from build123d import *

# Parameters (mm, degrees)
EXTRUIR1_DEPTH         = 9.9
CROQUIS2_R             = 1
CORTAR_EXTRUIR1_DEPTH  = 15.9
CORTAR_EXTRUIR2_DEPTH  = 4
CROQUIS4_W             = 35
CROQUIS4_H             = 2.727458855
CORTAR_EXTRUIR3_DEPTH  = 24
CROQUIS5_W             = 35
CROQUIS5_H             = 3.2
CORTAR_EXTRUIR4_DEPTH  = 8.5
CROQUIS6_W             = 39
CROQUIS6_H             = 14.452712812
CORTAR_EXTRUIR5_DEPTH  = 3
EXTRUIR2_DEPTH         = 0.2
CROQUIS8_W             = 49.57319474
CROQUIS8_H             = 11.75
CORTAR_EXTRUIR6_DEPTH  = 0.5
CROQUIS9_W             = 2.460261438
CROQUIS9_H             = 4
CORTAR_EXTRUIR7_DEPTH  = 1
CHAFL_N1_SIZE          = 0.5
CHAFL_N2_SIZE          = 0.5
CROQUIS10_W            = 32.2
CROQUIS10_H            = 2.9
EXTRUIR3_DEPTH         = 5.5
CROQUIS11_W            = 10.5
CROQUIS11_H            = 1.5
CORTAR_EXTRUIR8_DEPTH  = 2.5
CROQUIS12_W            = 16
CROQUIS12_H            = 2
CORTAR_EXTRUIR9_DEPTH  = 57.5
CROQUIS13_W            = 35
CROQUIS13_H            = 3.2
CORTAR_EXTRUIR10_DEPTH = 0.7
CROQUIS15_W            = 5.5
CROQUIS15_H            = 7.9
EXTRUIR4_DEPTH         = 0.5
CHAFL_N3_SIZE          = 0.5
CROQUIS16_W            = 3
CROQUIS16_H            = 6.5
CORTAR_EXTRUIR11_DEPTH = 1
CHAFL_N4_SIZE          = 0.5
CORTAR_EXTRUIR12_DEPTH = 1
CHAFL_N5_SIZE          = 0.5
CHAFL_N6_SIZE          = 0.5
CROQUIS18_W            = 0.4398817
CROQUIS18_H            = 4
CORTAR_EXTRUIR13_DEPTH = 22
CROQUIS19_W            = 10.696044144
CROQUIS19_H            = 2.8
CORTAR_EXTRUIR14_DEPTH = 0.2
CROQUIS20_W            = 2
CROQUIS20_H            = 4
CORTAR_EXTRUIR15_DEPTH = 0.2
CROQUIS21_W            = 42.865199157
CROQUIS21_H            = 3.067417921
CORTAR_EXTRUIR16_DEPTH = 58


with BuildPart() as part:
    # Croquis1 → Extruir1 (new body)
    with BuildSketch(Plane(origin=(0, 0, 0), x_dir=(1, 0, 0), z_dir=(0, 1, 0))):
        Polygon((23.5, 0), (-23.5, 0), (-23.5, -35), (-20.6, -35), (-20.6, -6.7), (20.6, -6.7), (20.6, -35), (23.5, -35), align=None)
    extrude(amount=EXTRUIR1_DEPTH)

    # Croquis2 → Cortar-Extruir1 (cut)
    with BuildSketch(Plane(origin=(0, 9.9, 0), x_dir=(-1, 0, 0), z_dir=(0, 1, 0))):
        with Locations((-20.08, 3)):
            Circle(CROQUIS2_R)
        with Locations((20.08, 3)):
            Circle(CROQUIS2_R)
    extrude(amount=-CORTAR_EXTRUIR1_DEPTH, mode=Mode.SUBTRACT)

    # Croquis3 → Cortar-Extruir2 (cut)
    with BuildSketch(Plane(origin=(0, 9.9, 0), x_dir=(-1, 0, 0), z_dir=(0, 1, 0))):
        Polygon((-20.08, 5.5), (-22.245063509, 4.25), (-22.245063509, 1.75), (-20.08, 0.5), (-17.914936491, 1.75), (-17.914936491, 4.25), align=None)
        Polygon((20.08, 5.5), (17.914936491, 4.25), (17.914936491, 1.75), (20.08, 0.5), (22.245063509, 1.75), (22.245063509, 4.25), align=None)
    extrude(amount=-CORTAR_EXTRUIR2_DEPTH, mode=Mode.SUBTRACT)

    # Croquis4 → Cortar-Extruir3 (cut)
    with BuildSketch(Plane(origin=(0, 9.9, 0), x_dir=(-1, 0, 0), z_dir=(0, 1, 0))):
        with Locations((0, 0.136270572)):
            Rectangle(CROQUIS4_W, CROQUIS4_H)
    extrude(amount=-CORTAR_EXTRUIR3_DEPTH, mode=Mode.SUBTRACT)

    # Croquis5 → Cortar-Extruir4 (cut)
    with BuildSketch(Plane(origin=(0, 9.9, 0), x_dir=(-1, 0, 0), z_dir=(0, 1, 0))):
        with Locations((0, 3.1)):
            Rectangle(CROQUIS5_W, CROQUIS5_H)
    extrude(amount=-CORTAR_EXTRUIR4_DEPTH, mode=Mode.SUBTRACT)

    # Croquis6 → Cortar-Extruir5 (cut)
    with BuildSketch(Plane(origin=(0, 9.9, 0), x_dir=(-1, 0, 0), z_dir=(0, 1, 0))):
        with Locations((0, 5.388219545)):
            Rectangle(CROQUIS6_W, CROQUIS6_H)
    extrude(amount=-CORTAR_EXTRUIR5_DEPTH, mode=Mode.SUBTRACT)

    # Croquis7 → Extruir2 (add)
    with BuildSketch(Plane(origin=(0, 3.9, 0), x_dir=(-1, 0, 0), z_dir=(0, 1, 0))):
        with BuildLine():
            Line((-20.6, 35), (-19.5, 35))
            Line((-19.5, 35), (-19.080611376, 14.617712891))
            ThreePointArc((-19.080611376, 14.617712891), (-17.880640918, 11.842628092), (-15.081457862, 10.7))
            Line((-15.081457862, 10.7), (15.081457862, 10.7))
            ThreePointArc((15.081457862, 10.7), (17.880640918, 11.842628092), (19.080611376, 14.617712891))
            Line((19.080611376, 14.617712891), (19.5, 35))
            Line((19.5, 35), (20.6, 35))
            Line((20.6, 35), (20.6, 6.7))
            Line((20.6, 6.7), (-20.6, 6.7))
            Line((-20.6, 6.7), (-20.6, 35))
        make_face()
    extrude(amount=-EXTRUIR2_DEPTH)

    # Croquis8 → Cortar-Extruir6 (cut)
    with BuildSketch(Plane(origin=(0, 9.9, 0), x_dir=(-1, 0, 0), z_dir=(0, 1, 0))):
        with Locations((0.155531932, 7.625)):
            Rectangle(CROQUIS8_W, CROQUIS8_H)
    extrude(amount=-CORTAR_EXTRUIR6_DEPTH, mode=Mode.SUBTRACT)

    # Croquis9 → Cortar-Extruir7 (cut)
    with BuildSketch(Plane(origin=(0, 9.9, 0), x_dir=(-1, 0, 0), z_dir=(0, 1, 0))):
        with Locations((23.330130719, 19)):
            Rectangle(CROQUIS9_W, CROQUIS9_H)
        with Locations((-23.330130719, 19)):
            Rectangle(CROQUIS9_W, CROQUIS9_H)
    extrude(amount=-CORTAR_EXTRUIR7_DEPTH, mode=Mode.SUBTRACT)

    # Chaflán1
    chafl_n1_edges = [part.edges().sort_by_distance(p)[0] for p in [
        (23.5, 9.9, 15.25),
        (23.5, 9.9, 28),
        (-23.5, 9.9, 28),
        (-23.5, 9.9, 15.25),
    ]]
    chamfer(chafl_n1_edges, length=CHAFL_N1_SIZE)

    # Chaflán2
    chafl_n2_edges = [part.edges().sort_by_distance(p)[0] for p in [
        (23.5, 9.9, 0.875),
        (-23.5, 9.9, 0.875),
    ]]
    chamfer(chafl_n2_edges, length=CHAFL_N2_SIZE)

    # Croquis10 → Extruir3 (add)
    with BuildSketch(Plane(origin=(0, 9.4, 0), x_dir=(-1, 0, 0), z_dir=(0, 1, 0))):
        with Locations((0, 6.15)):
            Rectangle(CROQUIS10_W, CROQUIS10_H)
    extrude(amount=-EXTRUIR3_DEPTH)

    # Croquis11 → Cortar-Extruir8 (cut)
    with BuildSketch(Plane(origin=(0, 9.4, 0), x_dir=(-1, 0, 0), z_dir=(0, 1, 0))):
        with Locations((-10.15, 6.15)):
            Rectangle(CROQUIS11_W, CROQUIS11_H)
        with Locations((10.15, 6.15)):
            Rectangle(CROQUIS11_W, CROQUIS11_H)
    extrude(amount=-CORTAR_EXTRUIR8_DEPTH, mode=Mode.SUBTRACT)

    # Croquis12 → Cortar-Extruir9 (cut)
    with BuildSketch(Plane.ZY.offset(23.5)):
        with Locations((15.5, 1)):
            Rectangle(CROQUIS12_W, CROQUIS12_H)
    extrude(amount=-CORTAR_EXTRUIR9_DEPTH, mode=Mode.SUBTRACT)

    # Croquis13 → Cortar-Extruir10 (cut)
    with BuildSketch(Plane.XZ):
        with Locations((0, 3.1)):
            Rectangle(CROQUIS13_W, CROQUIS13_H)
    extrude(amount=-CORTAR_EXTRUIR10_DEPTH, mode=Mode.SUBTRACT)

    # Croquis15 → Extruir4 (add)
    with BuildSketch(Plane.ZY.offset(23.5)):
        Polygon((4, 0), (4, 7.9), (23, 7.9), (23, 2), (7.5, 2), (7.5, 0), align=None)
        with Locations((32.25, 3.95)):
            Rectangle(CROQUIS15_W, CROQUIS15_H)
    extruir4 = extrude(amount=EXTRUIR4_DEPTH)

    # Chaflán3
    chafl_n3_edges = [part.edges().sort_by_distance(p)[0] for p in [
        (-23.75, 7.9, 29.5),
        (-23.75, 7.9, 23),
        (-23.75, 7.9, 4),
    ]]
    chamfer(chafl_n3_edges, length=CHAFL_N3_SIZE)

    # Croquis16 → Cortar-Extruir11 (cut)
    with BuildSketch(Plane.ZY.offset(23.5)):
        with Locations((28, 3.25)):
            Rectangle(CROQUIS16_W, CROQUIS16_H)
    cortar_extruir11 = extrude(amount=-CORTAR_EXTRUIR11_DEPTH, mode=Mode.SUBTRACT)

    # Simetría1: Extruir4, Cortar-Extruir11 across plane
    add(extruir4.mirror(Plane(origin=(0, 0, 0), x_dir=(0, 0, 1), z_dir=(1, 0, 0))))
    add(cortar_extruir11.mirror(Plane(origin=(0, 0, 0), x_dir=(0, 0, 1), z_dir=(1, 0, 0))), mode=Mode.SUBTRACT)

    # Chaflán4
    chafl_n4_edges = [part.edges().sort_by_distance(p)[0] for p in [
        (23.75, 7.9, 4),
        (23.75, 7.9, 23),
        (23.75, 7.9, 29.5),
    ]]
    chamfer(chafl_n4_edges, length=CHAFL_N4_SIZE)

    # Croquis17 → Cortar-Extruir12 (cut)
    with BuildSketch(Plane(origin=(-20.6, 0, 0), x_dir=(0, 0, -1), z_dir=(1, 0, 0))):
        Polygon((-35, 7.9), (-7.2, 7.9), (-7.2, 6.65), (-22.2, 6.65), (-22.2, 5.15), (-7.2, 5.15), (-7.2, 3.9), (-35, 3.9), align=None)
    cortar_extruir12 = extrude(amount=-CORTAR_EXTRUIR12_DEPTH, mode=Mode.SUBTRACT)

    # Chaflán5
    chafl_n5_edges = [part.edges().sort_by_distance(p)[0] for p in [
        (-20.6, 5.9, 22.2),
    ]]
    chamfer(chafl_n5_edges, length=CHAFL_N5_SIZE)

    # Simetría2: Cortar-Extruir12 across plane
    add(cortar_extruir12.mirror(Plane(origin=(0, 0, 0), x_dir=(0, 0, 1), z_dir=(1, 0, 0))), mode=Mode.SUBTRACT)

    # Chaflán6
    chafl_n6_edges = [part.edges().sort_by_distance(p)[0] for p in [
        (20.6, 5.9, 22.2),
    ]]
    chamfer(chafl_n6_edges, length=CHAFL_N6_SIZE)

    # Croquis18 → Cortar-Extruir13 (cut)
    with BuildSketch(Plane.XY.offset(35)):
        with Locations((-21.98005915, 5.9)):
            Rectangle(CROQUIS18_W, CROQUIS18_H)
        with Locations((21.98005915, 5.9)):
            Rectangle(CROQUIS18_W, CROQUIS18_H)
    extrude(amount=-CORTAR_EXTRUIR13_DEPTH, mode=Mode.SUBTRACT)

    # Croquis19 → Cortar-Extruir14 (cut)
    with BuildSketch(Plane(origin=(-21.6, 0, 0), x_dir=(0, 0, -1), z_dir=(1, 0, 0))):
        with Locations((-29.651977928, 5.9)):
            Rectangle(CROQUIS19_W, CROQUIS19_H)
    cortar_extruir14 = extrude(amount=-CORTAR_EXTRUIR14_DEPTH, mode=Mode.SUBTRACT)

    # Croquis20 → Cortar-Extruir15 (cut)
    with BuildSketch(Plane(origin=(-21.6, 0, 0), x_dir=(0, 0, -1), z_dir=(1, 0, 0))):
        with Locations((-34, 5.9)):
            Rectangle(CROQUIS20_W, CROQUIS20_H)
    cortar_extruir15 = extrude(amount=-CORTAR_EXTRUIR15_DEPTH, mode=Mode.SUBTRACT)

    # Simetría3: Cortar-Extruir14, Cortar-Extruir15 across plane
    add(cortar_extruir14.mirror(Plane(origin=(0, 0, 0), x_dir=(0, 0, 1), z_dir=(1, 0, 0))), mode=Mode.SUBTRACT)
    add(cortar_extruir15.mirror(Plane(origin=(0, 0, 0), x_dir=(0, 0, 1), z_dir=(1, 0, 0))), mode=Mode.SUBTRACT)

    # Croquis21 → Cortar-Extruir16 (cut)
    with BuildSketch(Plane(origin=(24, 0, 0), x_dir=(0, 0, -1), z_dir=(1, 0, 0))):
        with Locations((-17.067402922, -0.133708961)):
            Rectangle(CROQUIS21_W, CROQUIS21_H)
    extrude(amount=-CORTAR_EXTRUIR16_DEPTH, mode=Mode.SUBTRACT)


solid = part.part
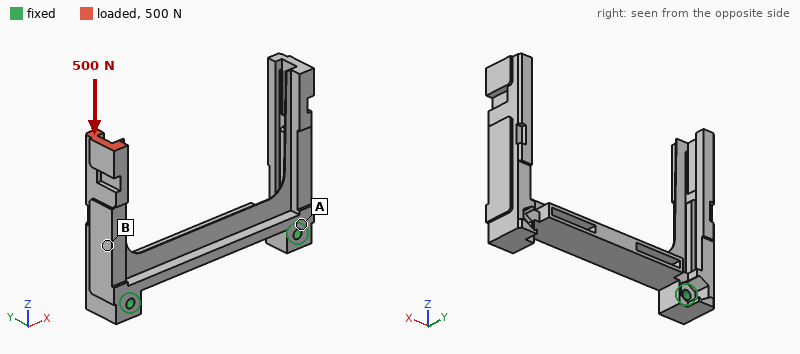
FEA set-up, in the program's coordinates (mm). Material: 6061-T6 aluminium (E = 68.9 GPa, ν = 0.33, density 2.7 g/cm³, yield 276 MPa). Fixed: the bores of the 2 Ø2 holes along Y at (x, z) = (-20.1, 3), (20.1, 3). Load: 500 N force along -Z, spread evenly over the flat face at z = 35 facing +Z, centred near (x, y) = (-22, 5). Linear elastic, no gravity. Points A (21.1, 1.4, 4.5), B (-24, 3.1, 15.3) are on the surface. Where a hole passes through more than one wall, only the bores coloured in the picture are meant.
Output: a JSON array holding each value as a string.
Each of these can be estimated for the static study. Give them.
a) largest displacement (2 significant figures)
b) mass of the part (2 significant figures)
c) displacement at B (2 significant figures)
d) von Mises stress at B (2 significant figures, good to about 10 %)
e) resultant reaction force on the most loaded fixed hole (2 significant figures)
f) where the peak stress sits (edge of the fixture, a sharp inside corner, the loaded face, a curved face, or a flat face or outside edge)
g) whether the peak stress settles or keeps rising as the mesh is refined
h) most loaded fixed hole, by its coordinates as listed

["72 µm", "6.2 g", "16 µm", "29 MPa", "500 N", "edge of the fixture", "keeps rising", "(-20.1, 3)"]
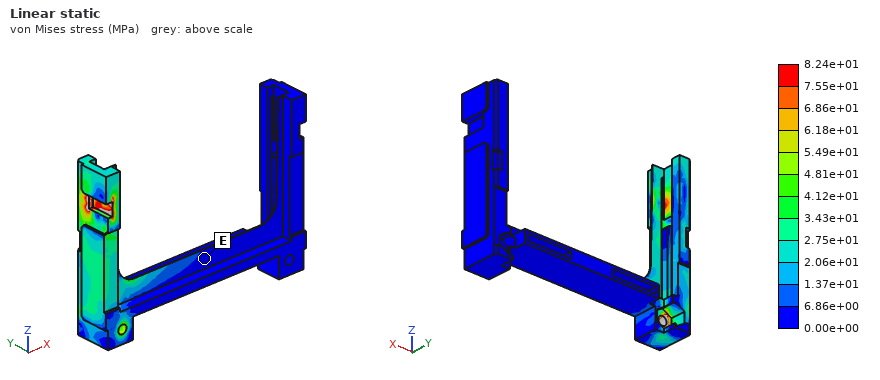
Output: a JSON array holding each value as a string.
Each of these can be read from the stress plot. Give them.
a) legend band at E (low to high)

["0.00e+00 to 6.86e+00 MPa"]
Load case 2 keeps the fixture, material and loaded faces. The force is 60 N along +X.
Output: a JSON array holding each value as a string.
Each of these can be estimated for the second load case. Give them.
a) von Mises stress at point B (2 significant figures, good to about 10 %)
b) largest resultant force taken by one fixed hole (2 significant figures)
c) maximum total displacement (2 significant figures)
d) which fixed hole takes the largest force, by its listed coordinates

["96 MPa", "91 N", "0.39 mm", "(20.1, 3)"]
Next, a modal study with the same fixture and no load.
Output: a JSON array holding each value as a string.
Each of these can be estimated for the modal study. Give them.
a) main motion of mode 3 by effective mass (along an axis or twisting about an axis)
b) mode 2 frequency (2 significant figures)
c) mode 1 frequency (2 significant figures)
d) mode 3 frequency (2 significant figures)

["along Y", "3300 Hz", "3300 Hz", "4900 Hz"]
